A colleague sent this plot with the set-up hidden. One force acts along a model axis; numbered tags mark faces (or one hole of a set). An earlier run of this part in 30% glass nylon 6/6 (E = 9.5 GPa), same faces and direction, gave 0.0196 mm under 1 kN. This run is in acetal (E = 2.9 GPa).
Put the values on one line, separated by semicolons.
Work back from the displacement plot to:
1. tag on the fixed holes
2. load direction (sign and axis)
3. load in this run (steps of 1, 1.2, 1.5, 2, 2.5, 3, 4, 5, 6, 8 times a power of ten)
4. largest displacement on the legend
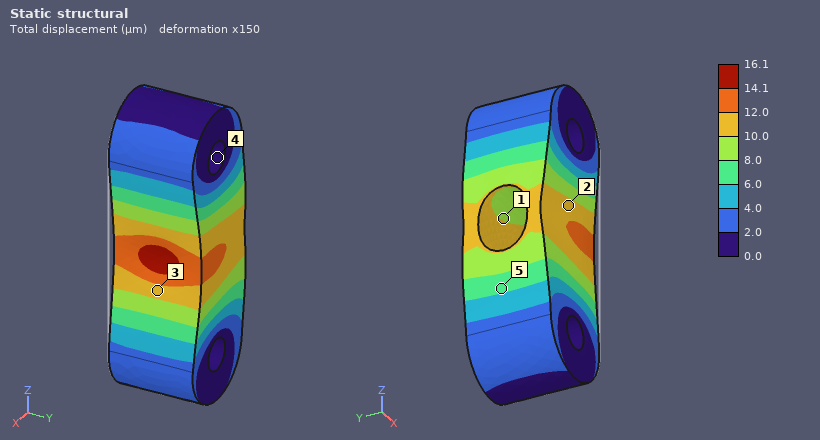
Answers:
4; -X; 250 N; 16.1 µm
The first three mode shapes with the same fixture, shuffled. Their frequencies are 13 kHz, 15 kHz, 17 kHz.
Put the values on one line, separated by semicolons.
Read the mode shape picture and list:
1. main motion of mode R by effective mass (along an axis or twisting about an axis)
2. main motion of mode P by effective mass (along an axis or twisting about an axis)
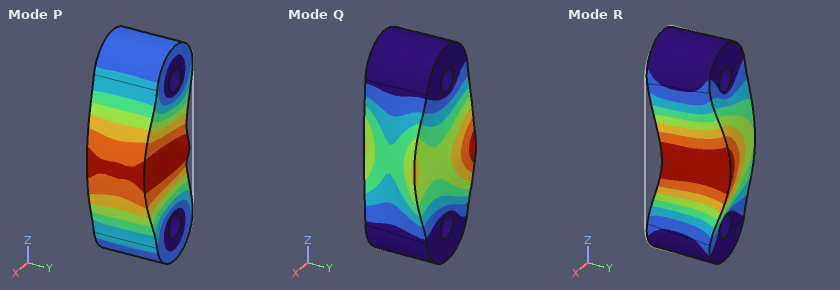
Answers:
along Y; along X
